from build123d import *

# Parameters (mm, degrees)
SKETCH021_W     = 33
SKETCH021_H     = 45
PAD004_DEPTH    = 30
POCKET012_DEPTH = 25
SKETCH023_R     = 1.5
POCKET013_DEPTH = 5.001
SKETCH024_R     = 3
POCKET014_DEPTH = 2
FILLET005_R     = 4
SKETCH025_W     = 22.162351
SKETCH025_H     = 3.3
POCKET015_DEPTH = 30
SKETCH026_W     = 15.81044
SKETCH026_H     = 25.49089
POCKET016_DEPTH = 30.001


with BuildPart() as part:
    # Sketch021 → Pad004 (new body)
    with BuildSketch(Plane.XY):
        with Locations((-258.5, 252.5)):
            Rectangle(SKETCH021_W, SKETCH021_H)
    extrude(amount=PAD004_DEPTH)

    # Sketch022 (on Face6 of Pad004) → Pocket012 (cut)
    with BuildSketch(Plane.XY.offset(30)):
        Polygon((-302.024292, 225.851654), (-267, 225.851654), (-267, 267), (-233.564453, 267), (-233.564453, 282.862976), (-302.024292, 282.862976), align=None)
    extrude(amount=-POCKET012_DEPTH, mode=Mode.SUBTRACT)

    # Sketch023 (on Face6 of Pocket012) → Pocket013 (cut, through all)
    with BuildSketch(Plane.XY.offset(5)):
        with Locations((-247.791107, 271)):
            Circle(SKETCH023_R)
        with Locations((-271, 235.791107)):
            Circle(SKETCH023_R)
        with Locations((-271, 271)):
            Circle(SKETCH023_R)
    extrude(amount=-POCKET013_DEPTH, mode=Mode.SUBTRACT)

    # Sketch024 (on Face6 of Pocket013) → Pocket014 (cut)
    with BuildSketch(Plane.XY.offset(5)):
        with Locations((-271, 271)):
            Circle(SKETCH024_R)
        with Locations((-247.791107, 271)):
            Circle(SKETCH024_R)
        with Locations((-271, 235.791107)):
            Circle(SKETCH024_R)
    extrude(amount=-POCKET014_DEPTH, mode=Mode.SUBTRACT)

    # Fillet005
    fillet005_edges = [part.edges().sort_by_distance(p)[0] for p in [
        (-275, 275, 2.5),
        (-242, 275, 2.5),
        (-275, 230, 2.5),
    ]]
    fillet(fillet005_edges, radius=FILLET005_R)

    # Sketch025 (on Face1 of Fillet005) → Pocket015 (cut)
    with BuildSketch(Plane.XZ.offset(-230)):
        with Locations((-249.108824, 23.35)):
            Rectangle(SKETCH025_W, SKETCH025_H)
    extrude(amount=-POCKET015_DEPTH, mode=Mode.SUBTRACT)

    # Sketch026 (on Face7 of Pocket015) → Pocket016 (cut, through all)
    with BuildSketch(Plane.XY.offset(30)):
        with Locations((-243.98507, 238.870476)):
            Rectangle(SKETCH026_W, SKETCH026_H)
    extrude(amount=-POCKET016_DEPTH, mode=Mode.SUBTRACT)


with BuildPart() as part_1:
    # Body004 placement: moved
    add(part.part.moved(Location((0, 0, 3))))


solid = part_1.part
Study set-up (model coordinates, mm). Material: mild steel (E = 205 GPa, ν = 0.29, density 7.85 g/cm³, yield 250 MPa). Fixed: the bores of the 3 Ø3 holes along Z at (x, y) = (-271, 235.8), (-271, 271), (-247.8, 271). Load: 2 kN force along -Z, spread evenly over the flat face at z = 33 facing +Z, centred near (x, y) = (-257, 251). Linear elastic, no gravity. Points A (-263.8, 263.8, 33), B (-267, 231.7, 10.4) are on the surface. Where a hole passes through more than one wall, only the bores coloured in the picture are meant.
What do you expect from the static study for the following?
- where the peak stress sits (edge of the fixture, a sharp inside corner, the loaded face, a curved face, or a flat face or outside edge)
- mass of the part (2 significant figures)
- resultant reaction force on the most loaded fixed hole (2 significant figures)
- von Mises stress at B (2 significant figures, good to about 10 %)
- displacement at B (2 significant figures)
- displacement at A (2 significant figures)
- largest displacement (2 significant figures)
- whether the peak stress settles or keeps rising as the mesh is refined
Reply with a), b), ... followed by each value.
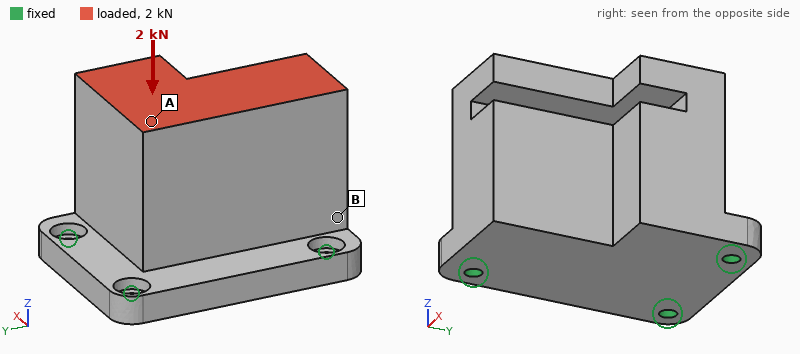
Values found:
a) edge of the fixture
b) 180 g
c) 1.2 kN
d) 27 MPa
e) 5.2 µm
f) 8.7 µm
g) 17 µm
h) keeps rising
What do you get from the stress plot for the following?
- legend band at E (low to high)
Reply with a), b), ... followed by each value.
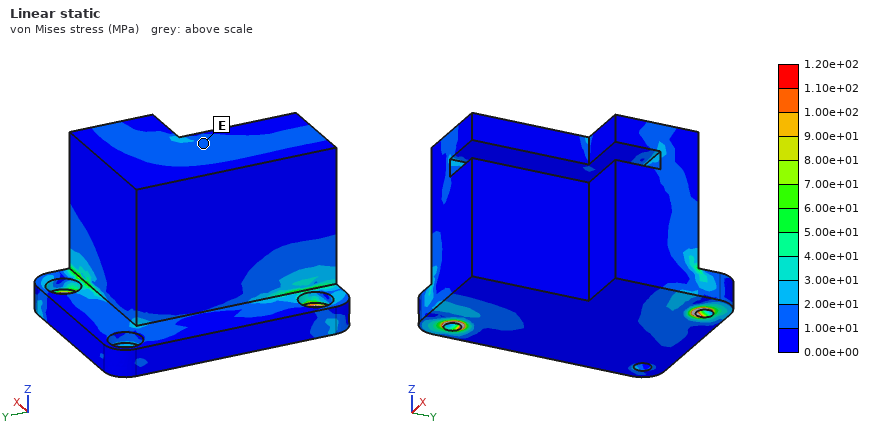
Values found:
a) 1.00e+01 to 2.00e+01 MPa
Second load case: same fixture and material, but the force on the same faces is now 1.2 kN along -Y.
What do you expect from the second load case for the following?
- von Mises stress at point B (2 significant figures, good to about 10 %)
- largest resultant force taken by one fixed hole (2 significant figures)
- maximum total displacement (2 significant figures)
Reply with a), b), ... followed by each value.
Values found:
a) 26 MPa
b) 1.2 kN
c) 17 µm
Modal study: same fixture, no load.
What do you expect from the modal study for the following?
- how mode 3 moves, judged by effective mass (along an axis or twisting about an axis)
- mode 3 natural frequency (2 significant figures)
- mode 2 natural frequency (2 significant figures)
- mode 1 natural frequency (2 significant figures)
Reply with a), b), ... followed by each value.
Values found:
a) along Z
b) 11 kHz
c) 9400 Hz
d) 4300 Hz
